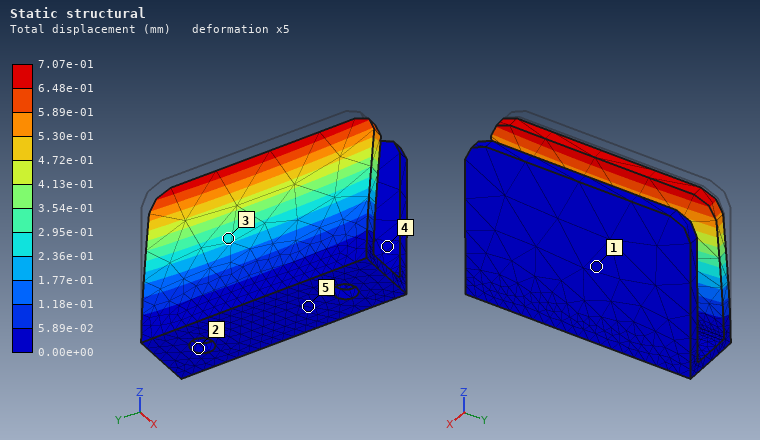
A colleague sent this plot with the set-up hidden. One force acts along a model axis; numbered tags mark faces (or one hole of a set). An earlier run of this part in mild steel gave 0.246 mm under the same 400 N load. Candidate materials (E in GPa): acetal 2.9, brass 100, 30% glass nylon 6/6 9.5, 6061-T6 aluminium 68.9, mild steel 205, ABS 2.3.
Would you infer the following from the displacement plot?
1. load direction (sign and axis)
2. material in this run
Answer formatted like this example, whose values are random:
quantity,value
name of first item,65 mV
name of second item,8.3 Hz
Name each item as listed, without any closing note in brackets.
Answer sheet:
quantity,value
load direction,+X
material in this run,6061-T6 aluminium
